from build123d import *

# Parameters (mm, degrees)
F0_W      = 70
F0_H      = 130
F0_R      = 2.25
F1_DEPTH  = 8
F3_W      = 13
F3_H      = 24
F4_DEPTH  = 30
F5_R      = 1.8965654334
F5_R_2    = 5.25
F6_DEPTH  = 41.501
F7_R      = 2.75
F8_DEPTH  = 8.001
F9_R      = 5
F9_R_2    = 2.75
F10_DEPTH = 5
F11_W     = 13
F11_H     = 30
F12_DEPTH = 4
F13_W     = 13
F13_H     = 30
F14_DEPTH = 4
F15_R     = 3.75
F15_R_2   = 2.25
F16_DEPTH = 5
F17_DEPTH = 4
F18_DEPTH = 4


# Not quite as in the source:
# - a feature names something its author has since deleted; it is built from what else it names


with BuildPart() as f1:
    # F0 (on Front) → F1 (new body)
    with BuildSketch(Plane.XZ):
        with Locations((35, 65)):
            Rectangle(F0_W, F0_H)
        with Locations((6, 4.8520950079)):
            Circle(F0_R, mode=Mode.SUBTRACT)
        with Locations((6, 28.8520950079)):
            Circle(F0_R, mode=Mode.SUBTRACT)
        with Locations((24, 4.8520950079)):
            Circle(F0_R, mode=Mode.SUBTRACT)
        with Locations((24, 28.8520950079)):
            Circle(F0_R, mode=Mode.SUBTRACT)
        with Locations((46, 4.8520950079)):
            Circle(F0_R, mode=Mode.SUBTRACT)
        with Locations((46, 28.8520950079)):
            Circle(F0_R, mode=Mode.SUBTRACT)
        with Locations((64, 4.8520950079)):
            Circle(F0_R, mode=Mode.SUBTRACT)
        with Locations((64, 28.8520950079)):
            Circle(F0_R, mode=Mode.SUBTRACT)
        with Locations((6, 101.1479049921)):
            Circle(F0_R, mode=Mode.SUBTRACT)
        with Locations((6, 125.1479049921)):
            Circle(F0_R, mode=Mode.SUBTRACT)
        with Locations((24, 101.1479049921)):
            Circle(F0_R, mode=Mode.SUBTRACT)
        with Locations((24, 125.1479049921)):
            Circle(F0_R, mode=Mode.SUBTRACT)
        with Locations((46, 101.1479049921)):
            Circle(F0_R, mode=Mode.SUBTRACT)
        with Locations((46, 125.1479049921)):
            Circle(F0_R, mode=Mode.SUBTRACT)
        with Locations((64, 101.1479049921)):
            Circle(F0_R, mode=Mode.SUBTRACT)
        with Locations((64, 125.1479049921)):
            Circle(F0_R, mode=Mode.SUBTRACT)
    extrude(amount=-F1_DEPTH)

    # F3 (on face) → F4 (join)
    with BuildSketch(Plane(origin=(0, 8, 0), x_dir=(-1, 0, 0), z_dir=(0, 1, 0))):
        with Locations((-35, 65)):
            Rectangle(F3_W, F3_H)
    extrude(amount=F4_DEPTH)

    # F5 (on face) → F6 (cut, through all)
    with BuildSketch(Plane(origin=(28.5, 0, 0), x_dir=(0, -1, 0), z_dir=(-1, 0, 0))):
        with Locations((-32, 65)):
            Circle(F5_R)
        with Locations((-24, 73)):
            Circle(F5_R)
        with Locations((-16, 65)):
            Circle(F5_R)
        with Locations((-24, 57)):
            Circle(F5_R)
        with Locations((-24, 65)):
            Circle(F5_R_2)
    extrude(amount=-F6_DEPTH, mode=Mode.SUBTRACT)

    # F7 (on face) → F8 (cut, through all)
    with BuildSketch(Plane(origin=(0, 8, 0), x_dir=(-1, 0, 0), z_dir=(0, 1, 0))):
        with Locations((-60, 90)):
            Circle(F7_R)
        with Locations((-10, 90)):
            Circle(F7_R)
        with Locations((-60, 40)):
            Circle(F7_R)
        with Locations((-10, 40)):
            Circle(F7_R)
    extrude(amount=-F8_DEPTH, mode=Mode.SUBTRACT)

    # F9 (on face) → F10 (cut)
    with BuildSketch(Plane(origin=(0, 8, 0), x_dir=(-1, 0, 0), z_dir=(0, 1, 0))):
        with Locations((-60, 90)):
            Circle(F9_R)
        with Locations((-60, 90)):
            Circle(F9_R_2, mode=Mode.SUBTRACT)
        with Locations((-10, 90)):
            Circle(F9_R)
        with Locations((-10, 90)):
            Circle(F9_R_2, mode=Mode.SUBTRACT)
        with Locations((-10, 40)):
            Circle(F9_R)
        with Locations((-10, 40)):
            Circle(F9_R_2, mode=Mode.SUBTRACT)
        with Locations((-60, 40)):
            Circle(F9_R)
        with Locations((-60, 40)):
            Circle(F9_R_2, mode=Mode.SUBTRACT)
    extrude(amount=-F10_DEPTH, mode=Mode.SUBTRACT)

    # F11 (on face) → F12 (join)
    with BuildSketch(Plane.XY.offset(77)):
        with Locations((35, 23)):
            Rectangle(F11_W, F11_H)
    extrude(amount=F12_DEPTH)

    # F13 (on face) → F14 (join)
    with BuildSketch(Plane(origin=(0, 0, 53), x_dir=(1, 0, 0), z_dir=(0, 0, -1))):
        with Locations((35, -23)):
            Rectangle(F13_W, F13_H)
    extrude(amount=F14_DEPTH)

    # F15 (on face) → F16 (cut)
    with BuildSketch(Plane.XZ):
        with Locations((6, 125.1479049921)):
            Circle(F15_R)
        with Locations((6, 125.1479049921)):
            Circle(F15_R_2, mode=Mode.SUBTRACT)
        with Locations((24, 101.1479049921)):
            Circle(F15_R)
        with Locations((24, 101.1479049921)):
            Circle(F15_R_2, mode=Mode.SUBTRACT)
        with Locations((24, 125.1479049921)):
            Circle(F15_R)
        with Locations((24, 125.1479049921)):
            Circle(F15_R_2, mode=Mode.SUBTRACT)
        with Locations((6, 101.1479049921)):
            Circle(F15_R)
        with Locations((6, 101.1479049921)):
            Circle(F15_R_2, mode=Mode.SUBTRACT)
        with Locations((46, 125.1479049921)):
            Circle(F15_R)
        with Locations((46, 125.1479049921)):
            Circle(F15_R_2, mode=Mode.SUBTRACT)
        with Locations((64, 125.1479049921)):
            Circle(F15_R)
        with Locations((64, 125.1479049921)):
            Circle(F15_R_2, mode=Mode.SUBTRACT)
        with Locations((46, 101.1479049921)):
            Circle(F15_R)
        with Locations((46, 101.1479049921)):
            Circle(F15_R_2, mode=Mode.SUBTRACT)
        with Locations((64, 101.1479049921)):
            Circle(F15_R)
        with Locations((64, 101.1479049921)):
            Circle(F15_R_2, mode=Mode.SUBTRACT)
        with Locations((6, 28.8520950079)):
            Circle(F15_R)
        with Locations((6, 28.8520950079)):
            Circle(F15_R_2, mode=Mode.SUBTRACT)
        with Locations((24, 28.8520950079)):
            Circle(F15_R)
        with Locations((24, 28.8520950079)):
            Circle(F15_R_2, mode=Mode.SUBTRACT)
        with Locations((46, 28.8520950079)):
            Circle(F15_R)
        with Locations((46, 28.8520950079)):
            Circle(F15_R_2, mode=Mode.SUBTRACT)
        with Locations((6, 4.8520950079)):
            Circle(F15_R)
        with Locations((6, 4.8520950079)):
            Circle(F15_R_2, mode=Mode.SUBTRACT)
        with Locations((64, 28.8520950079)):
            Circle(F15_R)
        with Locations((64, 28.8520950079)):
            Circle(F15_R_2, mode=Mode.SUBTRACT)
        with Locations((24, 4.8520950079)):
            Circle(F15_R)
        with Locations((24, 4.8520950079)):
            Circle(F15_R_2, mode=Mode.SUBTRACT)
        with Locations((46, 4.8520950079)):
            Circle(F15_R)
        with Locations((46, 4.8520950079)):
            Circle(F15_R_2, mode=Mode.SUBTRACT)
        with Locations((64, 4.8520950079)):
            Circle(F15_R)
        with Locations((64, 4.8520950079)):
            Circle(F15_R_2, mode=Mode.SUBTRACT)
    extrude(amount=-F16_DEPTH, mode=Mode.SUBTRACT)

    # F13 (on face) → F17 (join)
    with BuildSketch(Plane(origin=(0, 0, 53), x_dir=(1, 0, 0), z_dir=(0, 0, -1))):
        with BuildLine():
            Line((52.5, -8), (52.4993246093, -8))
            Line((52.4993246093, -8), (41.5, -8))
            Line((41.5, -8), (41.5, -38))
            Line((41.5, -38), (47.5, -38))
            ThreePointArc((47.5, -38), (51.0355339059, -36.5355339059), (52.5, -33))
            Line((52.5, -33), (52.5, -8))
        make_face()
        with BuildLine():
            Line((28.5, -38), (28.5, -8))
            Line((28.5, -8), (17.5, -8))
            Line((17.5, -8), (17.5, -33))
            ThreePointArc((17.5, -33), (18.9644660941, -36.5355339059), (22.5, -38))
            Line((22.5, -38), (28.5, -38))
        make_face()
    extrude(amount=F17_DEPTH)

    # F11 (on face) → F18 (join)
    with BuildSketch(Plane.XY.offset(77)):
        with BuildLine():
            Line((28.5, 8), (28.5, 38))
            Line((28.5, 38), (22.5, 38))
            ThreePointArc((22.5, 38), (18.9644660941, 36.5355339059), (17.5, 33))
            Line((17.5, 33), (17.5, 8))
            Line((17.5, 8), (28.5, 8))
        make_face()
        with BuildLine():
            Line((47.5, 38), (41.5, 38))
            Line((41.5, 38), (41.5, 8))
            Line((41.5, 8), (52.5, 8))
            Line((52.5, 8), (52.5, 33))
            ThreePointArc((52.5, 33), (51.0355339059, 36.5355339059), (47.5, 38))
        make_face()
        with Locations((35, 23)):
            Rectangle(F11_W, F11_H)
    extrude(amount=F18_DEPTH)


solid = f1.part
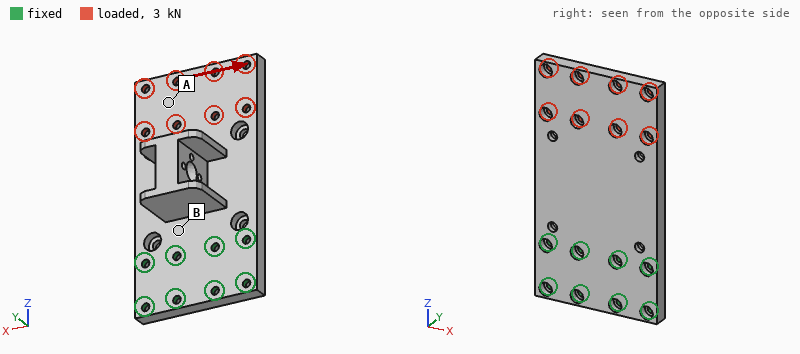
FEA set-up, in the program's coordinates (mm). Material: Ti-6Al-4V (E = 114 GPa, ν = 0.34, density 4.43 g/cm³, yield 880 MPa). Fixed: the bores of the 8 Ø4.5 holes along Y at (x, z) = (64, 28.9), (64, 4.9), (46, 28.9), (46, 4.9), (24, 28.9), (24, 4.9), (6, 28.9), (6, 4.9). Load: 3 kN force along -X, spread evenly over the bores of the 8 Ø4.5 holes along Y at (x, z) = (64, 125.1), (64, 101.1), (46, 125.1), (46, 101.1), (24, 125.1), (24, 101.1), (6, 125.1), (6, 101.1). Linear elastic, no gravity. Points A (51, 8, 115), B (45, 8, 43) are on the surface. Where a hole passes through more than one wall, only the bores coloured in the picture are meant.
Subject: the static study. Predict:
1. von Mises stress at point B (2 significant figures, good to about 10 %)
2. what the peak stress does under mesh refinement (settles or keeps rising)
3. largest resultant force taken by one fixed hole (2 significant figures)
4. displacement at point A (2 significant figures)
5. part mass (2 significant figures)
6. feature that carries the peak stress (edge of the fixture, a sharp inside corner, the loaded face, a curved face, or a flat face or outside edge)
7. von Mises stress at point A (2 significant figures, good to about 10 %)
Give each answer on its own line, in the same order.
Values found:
31 MPa
keeps rising
2.7 kN
58 µm
370 g
edge of the fixture
12 MPa
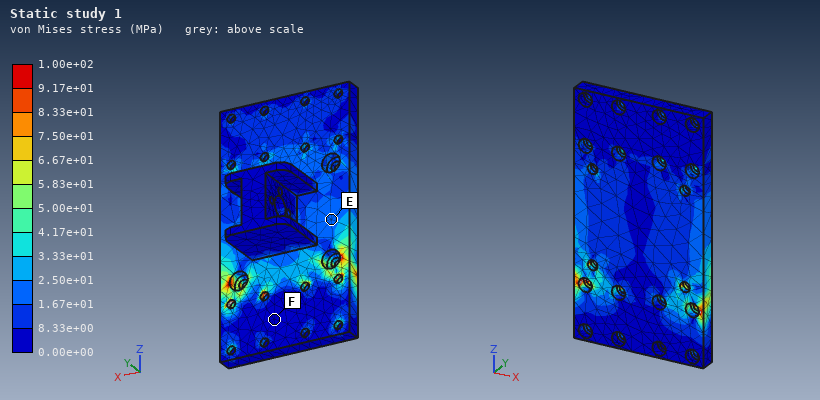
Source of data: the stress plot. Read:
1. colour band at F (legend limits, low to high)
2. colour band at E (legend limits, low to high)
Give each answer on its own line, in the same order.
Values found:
0.00e+00 to 8.33e+00 MPa
1.67e+01 to 2.50e+01 MPa
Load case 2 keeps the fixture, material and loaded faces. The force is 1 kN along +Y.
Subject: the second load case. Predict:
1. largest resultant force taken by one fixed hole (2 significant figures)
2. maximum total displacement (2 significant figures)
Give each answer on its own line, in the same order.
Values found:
2.5 kN
0.84 mm
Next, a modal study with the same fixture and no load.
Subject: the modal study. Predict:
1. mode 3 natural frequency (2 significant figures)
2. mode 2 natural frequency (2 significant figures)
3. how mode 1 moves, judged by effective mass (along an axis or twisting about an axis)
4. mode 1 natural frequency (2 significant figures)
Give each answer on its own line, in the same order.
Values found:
3400 Hz
2200 Hz
along Y
590 Hz
